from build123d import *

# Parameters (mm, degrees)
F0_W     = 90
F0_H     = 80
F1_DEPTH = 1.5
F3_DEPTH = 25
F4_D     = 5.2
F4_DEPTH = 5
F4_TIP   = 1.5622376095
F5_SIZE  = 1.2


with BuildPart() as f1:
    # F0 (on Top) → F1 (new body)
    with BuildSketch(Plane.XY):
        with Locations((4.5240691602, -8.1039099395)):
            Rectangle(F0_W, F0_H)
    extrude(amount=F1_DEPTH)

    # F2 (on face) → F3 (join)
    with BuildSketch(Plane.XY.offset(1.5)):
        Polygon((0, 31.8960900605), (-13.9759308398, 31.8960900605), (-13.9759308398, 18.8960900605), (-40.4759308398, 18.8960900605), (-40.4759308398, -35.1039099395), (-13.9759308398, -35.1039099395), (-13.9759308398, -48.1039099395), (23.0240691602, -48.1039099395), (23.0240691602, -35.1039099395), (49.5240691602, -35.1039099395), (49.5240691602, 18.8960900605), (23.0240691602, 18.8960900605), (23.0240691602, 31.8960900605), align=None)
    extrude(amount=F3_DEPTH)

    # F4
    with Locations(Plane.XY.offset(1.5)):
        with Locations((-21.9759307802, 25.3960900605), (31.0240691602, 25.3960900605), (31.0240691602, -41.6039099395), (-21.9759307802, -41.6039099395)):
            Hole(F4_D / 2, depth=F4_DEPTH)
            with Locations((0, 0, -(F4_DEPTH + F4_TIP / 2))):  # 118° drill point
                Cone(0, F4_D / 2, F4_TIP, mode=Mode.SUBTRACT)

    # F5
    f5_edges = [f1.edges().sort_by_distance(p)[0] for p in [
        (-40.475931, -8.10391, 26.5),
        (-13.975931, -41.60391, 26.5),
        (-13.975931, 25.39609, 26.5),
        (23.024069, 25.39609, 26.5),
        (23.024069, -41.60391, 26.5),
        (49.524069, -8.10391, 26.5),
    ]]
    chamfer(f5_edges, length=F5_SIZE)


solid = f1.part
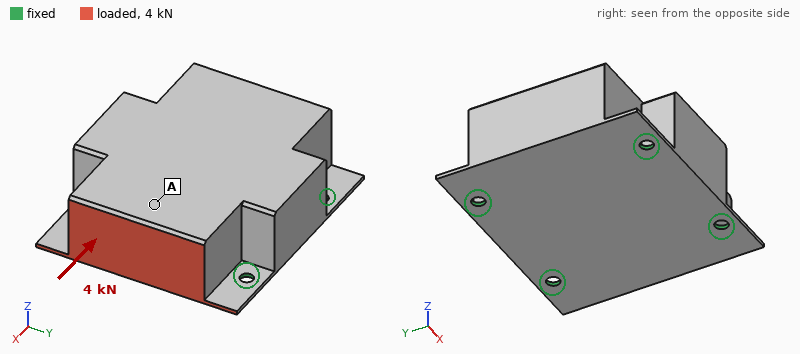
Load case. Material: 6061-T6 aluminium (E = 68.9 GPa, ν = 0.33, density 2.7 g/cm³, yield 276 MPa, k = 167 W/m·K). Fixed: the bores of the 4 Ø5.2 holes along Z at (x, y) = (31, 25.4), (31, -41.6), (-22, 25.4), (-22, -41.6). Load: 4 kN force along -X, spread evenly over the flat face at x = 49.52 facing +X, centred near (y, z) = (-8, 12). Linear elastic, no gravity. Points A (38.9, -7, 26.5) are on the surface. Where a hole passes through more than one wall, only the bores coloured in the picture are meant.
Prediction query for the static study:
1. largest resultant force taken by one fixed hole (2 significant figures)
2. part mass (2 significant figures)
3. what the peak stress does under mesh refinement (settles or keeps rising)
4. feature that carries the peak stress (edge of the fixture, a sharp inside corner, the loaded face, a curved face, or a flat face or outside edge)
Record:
1.2 kN
420 g
keeps rising
edge of the fixture
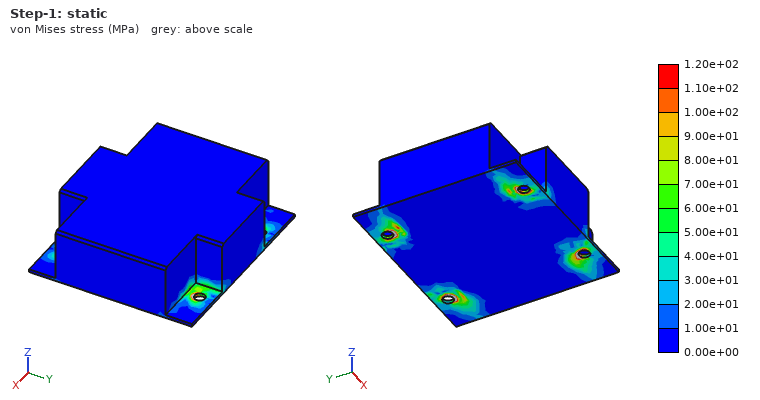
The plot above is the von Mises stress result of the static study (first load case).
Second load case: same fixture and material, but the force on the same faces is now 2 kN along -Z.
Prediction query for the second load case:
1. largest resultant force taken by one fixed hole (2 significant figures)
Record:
1.5 kN
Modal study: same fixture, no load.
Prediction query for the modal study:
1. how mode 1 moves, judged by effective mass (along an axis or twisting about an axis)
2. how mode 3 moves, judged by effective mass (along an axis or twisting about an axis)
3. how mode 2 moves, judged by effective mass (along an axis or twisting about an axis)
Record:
along X
along Y
along Z
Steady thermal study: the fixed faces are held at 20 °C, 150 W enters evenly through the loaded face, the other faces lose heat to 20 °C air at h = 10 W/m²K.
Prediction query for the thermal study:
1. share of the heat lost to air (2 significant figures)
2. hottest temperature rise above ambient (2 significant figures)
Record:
5.9 %
63 K
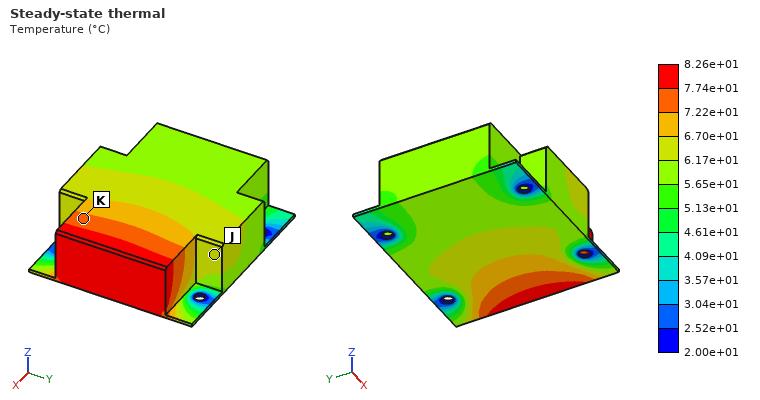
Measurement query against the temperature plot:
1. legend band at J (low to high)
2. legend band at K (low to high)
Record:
6.17e+01 to 6.70e+01 °C
7.22e+01 to 7.74e+01 °C
